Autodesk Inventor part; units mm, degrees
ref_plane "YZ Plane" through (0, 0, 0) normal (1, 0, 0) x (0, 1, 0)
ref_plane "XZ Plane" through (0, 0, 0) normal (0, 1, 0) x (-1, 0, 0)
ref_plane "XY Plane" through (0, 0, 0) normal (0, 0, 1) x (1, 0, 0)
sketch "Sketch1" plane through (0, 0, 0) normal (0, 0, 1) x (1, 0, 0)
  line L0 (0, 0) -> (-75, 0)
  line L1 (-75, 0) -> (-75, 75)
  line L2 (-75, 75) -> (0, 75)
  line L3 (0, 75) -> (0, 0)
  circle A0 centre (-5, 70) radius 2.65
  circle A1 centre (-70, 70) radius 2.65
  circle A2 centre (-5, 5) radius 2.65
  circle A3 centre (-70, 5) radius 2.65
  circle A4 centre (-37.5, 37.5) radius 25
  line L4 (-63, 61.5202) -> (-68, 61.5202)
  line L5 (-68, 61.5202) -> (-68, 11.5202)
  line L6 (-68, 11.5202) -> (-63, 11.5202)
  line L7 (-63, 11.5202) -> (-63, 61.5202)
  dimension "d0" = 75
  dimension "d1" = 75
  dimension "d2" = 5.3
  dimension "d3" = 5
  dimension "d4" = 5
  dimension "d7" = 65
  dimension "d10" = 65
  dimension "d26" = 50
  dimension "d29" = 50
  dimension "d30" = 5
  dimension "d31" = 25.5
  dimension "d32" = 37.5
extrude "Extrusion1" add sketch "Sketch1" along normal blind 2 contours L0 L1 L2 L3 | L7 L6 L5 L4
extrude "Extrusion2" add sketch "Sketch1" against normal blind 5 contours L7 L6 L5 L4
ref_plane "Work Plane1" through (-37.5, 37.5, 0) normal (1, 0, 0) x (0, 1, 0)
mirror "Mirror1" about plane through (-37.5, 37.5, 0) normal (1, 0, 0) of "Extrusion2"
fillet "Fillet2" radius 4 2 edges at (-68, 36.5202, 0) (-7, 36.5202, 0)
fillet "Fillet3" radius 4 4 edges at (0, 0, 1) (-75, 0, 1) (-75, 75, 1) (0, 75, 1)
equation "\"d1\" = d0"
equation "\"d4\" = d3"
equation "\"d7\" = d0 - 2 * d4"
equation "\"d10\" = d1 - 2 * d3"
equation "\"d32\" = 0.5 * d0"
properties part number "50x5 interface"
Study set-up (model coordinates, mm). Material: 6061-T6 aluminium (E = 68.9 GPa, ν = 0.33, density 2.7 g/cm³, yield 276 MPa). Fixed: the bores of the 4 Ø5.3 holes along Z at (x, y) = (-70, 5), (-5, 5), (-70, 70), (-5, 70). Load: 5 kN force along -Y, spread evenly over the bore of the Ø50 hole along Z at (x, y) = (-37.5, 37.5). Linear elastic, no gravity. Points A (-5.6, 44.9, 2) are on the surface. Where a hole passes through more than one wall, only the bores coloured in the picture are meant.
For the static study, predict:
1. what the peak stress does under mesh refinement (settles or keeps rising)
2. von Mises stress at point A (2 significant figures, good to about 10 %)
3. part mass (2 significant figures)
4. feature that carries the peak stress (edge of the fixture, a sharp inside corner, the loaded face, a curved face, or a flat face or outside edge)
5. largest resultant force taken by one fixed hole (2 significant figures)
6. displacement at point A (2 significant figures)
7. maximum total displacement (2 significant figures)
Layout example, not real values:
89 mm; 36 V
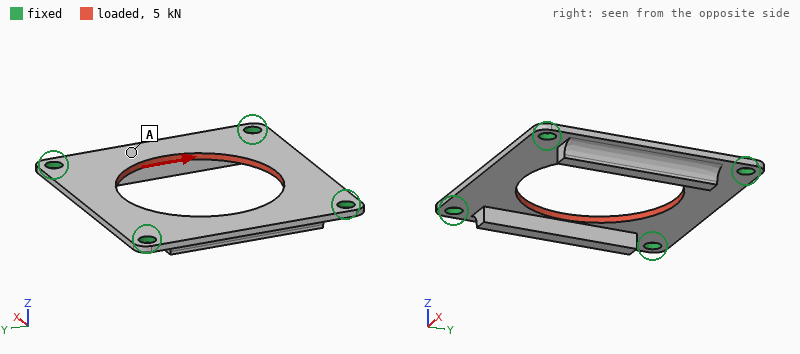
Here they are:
keeps rising; 30 MPa; 27 g; edge of the fixture; 1.3 kN; 13 µm; 47 µm
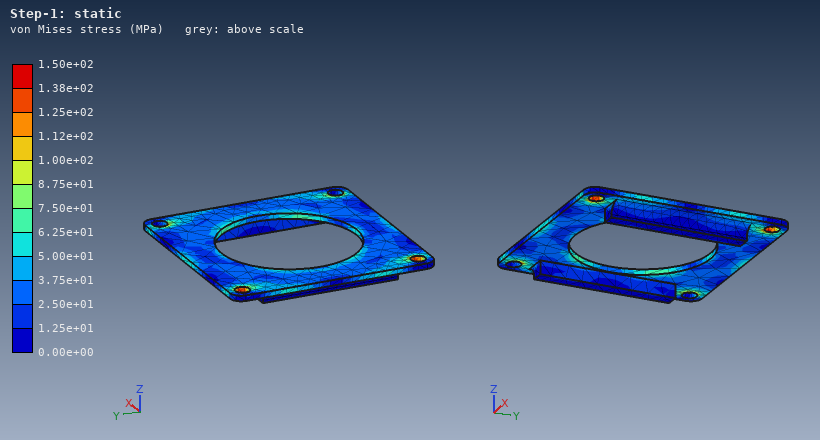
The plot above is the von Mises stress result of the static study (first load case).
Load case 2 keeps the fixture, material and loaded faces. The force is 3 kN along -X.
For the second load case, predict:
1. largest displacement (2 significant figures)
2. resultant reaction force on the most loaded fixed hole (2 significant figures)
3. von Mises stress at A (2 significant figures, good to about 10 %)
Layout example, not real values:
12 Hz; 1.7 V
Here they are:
29 µm; 790 N; 14 MPa
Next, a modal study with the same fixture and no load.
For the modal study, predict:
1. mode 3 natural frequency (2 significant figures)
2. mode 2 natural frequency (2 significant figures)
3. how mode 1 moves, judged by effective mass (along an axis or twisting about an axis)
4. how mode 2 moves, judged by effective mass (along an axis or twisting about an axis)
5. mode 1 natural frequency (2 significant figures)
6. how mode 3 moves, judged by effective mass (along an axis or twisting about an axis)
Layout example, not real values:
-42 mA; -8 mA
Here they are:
4800 Hz; 3300 Hz; along Z; twisting about X; 2900 Hz; along Z
